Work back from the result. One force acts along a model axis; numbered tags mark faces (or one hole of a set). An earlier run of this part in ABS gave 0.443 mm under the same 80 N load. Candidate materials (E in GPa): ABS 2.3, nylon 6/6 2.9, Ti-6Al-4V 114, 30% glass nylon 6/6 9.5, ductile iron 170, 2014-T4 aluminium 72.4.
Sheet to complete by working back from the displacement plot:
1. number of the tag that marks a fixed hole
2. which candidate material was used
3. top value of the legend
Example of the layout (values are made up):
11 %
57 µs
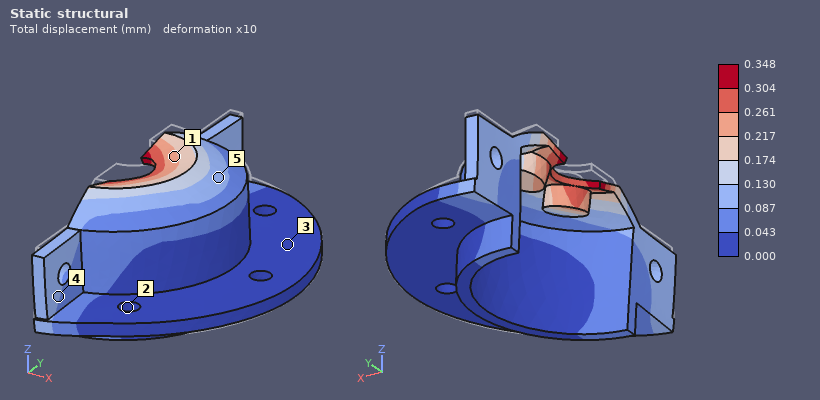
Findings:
2
nylon 6/6
0.348 mm
